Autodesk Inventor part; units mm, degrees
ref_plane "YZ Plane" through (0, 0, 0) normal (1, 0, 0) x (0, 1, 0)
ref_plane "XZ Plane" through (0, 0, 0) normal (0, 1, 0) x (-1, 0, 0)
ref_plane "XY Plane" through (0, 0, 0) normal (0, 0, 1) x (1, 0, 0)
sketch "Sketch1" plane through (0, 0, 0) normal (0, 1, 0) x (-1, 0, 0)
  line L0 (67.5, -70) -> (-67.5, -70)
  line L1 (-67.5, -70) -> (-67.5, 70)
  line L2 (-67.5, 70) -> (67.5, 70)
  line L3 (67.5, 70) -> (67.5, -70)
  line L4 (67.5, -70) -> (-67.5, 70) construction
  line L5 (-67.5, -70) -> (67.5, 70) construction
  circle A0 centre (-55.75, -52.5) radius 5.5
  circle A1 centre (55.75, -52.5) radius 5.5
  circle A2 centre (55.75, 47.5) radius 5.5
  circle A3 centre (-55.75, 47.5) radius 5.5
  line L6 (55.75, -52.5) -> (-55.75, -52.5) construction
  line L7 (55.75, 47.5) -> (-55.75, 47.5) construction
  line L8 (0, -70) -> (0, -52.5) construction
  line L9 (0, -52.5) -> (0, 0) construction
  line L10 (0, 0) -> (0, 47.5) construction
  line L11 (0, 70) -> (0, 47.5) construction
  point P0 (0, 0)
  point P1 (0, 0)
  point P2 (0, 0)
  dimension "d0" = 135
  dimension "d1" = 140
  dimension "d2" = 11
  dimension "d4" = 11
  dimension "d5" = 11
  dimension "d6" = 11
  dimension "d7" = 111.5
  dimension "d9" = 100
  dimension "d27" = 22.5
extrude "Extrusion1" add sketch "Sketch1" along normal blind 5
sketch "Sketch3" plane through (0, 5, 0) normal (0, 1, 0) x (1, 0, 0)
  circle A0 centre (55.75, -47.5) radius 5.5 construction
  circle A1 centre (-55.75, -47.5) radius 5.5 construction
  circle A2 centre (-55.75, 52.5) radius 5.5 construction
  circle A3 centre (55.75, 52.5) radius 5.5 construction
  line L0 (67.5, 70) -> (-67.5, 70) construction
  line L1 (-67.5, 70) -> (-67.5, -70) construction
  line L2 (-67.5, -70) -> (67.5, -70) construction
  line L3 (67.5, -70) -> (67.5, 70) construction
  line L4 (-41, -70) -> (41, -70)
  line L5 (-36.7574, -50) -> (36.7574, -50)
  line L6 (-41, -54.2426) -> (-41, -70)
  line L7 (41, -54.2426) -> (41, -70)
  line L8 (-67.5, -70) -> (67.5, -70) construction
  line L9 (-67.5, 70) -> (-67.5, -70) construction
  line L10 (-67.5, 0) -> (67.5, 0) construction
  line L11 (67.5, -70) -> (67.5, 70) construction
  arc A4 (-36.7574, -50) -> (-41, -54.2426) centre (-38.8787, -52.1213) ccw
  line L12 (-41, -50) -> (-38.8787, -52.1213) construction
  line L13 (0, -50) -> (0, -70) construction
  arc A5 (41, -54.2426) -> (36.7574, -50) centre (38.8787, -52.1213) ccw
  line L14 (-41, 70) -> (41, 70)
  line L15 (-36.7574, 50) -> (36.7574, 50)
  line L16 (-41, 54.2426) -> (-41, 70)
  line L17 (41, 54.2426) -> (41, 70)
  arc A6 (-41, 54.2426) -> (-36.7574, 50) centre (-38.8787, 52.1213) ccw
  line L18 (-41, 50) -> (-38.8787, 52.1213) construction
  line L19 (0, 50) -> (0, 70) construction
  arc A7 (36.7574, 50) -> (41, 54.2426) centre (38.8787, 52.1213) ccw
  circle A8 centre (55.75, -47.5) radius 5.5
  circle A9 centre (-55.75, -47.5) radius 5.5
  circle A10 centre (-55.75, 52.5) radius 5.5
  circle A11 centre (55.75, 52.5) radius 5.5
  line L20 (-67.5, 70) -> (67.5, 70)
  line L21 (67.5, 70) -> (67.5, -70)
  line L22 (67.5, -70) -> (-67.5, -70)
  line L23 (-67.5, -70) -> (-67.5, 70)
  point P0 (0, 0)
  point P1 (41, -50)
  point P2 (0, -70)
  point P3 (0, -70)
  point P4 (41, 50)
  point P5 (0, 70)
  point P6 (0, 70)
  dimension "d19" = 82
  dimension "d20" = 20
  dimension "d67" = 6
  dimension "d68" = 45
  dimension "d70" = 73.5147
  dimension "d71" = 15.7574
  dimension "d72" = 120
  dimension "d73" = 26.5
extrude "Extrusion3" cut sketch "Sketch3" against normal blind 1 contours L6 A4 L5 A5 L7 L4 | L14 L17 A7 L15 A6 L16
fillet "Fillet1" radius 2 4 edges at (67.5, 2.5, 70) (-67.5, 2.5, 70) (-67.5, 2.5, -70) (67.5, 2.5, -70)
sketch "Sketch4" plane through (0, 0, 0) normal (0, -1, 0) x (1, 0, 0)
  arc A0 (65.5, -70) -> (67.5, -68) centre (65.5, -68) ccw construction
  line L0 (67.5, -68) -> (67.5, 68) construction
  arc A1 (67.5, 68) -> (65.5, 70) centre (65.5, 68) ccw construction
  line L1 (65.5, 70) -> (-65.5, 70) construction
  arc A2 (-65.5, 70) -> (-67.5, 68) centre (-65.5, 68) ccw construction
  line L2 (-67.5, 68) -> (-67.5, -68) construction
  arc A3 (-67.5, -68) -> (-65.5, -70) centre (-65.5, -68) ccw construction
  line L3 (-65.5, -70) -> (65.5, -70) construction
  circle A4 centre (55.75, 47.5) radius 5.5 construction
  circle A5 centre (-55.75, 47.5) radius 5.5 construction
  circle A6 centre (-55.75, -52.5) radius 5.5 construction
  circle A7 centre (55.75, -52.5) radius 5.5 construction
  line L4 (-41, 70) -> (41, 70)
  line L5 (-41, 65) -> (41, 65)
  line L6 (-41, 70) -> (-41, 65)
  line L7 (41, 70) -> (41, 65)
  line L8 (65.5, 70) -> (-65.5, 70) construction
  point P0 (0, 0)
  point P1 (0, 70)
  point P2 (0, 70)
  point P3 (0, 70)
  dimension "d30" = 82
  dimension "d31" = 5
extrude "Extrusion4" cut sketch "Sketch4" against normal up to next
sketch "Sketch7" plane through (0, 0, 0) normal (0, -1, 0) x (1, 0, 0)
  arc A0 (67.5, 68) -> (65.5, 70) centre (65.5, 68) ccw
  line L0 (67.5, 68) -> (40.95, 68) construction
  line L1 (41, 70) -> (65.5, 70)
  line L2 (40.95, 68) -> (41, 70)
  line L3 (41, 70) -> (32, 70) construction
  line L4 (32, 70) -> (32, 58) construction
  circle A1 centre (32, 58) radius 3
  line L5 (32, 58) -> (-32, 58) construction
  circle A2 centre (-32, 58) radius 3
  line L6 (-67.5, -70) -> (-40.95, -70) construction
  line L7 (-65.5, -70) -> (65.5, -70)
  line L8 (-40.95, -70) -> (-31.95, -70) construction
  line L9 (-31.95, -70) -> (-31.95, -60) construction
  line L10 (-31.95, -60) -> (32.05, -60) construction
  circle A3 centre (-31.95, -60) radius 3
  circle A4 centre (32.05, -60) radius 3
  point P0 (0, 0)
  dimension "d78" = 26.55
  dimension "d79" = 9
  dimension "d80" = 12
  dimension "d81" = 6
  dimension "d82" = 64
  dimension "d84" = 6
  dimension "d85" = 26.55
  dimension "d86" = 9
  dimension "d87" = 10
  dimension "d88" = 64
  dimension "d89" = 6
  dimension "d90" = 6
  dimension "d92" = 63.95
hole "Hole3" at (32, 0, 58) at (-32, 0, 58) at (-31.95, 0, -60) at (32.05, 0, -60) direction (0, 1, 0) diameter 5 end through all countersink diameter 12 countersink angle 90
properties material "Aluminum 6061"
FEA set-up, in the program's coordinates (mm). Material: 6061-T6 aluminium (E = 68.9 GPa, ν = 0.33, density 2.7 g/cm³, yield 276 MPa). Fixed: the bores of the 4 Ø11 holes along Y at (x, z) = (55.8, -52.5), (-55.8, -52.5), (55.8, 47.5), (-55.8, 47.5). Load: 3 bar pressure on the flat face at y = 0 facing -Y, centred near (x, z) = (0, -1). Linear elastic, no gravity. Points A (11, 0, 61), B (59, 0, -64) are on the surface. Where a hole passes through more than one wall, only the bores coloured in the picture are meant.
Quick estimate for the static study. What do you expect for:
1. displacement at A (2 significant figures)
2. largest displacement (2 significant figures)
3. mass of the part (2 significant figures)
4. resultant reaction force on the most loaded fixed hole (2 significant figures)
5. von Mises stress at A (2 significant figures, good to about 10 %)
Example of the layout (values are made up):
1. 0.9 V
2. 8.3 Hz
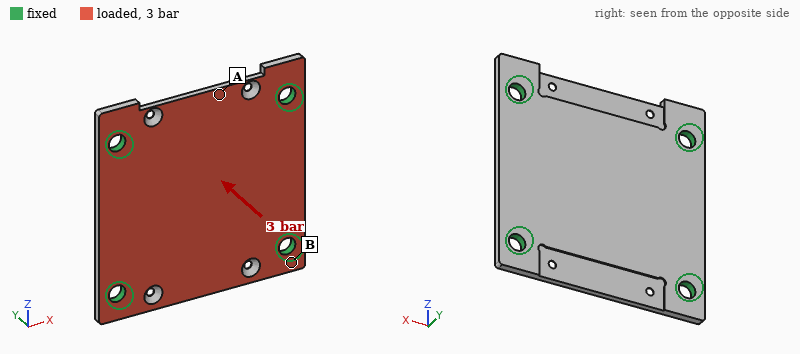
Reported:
1. 0.15 mm
2. 0.29 mm
3. 230 g
4. 1.4 kN
5. 37 MPa
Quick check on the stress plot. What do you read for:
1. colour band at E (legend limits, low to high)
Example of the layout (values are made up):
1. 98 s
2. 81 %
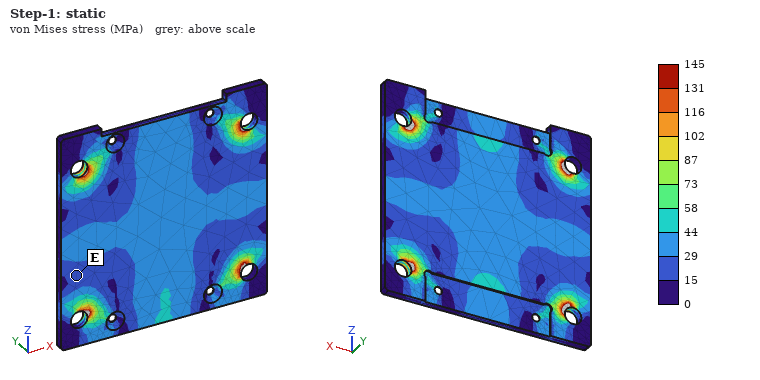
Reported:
1. 15 to 29 MPa
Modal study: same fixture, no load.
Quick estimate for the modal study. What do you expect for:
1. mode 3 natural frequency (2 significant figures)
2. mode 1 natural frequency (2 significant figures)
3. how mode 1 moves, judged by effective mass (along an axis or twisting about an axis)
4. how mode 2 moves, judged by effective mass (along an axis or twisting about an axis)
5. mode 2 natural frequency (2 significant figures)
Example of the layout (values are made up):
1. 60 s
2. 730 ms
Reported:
1. 2900 Hz
2. 1700 Hz
3. along Y
4. twisting about X
5. 2500 Hz
